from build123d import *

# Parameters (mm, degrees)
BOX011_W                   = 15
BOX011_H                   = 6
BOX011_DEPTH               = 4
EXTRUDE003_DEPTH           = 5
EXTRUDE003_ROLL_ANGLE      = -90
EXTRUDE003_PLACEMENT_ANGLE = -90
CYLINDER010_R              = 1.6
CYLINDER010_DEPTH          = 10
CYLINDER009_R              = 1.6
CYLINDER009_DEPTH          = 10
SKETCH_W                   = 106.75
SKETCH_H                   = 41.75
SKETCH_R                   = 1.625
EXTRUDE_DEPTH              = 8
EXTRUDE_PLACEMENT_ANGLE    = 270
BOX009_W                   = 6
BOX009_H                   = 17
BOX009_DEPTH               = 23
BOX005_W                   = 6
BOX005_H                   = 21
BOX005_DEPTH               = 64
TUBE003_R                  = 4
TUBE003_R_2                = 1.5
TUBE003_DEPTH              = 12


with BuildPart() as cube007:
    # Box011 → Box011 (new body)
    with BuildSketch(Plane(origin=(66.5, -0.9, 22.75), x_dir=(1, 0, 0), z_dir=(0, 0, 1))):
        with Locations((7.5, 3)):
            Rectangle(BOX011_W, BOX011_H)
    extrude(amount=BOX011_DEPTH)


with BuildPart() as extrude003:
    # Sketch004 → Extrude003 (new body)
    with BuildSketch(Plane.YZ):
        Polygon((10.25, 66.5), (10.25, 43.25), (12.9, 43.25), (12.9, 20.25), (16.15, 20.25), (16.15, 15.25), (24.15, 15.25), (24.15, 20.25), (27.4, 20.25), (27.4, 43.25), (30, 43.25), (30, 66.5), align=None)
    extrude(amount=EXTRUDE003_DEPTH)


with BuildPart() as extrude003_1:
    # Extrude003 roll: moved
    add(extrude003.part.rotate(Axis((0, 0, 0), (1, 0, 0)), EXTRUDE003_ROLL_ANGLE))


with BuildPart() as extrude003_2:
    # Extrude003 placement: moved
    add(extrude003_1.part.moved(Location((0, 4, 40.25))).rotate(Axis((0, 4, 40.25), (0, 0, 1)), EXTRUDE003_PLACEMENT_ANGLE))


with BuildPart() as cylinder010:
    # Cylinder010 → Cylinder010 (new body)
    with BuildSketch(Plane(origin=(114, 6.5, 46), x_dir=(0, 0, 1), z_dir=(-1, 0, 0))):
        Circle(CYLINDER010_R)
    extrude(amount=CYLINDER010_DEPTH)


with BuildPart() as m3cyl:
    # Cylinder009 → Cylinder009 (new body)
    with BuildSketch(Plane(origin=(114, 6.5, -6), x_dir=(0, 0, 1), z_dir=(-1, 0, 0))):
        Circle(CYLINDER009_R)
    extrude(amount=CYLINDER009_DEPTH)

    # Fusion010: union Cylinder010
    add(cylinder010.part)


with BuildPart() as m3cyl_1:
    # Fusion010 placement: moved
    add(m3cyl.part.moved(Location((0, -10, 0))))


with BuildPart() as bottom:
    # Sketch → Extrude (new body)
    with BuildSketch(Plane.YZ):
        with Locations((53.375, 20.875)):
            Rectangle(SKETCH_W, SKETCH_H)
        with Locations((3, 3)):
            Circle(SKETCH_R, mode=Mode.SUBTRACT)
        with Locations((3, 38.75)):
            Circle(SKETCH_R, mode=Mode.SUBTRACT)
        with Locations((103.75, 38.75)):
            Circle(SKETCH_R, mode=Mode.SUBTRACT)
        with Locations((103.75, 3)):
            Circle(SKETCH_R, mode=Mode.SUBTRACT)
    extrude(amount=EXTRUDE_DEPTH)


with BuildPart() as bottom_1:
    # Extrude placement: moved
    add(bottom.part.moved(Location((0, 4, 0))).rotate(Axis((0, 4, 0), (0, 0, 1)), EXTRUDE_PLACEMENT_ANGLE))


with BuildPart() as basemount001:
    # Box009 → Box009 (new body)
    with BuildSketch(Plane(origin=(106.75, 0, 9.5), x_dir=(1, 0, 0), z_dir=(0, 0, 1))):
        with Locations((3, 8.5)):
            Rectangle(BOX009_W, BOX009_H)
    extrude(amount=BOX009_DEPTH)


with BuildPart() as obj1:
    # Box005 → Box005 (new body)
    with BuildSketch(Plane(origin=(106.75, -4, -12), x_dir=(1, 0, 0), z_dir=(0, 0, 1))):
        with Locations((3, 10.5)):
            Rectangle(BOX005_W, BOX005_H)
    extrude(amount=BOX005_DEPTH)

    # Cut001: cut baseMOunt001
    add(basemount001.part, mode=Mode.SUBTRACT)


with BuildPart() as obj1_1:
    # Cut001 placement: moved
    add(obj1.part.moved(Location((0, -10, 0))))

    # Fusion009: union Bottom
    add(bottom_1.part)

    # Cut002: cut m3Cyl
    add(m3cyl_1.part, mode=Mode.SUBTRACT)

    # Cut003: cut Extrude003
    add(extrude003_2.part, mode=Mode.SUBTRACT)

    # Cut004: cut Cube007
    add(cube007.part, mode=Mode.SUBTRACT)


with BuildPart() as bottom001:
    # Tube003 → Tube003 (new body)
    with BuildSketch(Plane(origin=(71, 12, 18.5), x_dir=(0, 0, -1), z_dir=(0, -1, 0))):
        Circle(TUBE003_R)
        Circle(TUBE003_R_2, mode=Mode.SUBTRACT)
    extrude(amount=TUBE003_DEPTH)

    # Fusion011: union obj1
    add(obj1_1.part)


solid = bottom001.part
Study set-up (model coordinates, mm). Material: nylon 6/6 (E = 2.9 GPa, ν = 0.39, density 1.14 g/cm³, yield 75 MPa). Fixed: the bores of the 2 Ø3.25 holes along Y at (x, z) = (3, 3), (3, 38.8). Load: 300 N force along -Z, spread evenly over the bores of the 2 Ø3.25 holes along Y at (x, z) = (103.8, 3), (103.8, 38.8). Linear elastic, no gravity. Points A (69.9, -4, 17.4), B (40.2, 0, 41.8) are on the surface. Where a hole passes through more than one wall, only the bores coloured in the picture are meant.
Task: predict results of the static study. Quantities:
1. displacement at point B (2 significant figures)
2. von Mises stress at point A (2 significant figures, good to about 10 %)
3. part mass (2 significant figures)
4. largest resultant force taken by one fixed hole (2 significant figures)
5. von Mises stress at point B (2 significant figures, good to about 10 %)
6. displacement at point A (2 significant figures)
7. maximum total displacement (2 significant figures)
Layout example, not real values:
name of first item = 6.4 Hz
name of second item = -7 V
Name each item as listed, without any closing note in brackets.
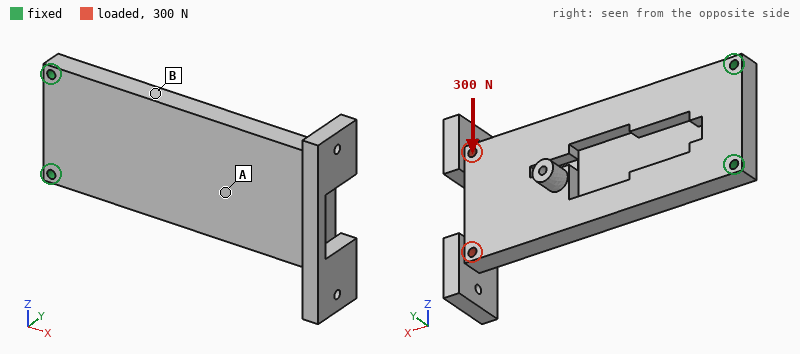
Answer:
displacement at point B = 0.29 mm
von Mises stress at point A = 2.7 MPa
part mass = 42 g
largest resultant force taken by one fixed hole = 860 N
von Mises stress at point B = 9.1 MPa
displacement at point A = 0.51 mm
maximum total displacement = 1.3 mm
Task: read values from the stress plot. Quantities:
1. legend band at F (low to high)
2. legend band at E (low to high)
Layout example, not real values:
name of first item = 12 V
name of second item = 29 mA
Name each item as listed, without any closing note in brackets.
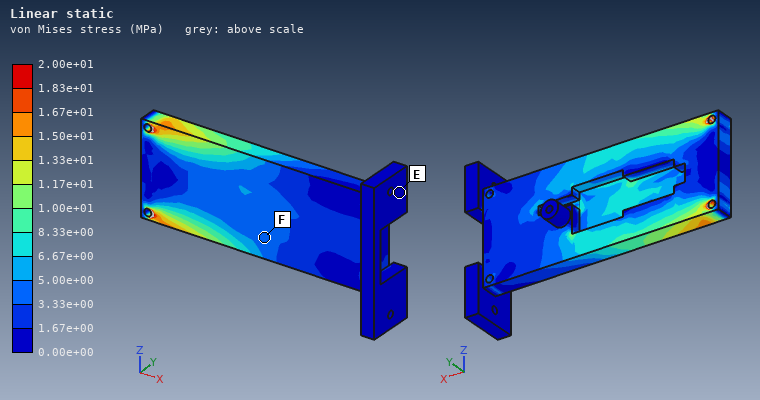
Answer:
legend band at F = 3.33e+00 to 5.00e+00 MPa
legend band at E = 0.00e+00 to 1.67e+00 MPa
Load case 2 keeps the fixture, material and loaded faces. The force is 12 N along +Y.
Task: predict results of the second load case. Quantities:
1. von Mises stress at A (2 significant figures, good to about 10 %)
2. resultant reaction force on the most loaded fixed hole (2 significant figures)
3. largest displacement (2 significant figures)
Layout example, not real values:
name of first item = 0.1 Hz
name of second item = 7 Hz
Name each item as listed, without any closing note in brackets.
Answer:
von Mises stress at A = 0.99 MPa
resultant reaction force on the most loaded fixed hole = 9.0 N
largest displacement = 1.3 mm
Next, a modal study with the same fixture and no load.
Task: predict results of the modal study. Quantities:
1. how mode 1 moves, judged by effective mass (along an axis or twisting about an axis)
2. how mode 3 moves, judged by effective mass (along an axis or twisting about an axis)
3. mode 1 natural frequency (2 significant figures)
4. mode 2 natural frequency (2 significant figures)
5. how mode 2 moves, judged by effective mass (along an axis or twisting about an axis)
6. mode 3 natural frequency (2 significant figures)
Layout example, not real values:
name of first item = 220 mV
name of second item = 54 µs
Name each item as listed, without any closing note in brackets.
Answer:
how mode 1 moves, judged by effective mass = along Y
how mode 3 moves, judged by effective mass = along Z
mode 1 natural frequency = 120 Hz
mode 2 natural frequency = 460 Hz
how mode 2 moves, judged by effective mass = twisting about X
mode 3 natural frequency = 650 Hz
